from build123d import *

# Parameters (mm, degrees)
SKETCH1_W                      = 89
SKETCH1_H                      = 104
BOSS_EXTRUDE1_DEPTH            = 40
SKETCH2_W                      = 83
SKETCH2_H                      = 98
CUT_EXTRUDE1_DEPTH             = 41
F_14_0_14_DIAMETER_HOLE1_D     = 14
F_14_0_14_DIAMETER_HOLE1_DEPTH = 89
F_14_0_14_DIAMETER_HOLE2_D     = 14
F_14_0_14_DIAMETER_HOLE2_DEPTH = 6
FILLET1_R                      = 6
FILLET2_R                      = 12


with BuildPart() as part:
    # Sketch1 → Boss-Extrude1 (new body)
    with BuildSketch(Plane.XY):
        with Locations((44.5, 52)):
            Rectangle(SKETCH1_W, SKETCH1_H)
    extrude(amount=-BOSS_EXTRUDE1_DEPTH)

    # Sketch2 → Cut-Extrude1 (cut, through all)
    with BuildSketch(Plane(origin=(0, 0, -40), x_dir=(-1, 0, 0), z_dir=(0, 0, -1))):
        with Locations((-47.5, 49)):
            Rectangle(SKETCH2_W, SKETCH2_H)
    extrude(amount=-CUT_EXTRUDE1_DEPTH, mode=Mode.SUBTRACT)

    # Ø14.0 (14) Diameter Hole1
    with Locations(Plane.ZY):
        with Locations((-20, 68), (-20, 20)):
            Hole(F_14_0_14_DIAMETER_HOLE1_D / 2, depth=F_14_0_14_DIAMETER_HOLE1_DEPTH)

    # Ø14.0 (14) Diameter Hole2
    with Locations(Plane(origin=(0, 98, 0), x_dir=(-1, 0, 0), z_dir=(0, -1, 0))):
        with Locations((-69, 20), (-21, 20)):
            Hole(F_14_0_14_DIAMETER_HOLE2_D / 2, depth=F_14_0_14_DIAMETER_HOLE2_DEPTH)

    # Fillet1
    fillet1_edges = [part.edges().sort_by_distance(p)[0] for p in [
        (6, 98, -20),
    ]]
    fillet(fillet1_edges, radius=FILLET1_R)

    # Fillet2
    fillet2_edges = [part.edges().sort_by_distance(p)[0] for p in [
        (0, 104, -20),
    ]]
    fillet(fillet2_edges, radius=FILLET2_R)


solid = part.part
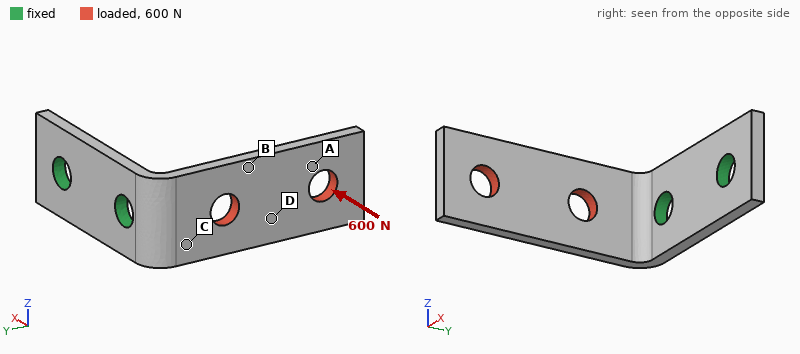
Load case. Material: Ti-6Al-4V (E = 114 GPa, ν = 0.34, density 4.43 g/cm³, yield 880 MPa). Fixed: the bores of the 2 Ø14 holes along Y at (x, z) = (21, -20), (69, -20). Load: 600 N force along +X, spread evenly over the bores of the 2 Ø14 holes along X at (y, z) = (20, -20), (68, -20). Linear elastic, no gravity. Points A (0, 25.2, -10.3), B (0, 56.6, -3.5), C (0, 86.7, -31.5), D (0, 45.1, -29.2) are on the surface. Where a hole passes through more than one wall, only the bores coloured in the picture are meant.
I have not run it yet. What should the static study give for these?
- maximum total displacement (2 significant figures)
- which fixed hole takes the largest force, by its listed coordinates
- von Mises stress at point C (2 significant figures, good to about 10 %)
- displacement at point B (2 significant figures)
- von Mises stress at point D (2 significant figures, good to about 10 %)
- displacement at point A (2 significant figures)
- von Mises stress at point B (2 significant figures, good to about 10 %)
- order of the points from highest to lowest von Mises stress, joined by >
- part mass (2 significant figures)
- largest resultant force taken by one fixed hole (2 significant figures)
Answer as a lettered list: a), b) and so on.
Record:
a) 1.5 mm
b) (21, -20)
c) 100 MPa
d) 0.49 mm
e) 33 MPa
f) 1.1 mm
g) 55 MPa
h) C > B > D > A
i) 180 g
j) 620 N
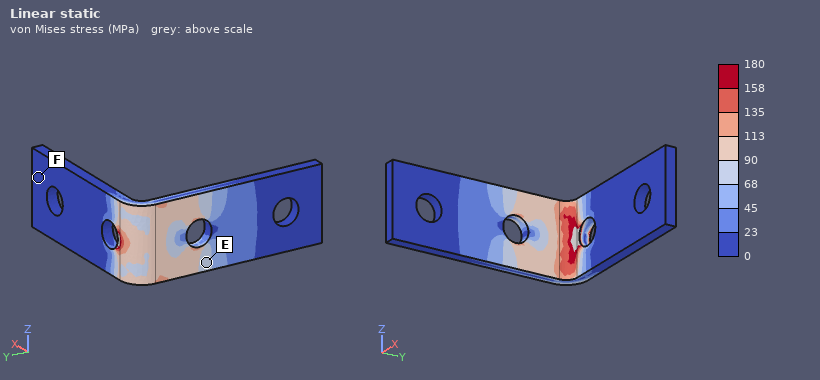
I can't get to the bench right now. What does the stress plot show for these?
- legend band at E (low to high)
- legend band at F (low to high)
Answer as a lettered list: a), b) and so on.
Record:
a) 68 to 90 MPa
b) 0 to 23 MPa
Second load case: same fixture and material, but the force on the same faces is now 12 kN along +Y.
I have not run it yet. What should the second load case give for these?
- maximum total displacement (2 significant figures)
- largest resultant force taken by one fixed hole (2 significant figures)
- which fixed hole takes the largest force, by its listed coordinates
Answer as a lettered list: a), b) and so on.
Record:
a) 1.5 mm
b) 12 kN
c) (21, -20)
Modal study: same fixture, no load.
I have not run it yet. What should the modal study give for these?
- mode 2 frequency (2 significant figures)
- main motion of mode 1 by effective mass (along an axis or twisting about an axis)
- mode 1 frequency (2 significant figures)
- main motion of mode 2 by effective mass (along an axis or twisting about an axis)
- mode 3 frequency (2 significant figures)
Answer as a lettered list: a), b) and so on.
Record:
a) 980 Hz
b) along X
c) 420 Hz
d) along Z
e) 2200 Hz
